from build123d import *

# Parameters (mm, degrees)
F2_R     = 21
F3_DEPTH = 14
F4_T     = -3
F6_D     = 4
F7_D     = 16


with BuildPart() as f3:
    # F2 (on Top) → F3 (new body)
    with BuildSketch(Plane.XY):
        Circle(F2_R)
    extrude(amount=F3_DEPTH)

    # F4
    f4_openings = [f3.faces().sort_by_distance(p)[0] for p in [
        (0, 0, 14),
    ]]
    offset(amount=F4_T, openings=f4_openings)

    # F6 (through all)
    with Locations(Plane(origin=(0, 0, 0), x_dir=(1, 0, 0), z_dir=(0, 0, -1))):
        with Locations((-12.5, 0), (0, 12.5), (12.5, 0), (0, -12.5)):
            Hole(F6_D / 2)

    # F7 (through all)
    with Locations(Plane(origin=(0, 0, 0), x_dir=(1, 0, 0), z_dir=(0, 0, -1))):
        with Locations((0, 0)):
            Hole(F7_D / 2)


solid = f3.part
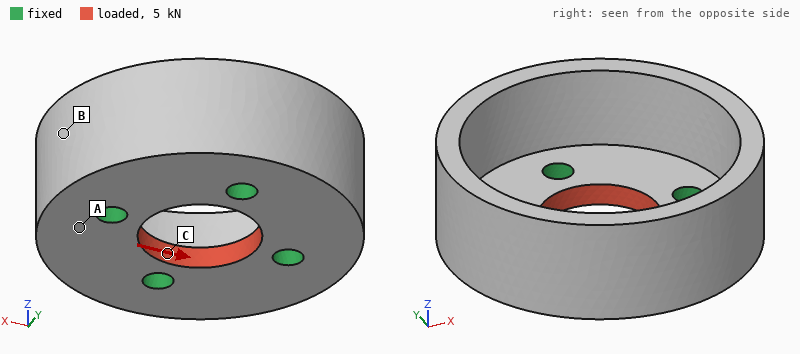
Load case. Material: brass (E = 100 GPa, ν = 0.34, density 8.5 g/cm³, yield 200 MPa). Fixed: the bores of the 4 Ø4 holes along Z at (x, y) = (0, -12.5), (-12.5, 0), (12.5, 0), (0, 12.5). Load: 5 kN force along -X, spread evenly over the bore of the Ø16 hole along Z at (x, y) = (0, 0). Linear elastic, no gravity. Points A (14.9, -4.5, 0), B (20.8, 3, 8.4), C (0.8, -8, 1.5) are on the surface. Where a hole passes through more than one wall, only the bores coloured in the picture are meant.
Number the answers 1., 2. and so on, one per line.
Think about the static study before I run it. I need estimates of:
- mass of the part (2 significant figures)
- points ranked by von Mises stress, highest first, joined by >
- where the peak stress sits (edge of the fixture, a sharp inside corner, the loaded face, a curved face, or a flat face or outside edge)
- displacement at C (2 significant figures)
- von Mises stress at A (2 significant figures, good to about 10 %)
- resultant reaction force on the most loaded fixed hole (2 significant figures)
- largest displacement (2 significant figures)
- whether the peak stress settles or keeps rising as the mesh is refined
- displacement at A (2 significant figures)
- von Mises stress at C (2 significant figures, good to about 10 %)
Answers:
1. 63 g
2. C > A > B
3. edge of the fixture
4. 3.0 µm
5. 17 MPa
6. 1.3 kN
7. 3.5 µm
8. keeps rising
9. 0.94 µm
10. 57 MPa
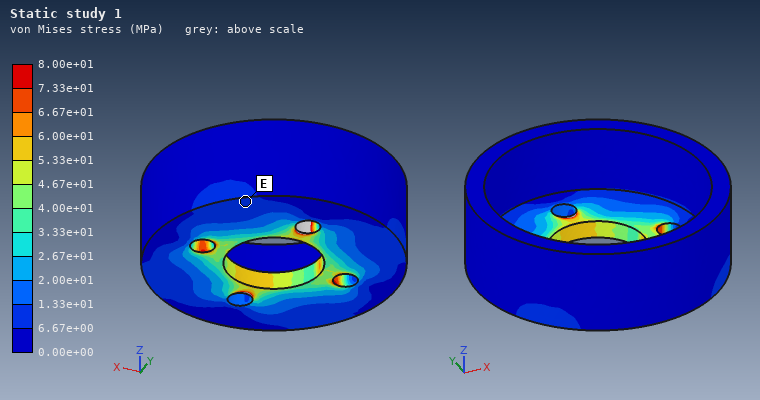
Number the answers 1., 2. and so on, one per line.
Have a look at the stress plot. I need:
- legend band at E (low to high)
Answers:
1. 6.67e+00 to 1.33e+01 MPa
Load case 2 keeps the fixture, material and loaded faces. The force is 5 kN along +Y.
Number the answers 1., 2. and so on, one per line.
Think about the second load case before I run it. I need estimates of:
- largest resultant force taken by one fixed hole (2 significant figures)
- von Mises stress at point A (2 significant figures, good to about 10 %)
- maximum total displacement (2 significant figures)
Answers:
1. 1.3 kN
2. 14 MPa
3. 3.5 µm
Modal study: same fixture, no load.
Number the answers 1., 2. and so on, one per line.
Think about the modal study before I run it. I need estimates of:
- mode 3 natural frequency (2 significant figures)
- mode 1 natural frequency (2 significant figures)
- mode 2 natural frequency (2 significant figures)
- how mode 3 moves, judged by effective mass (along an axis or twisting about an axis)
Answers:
1. 9300 Hz
2. 6800 Hz
3. 8700 Hz
4. along Y
